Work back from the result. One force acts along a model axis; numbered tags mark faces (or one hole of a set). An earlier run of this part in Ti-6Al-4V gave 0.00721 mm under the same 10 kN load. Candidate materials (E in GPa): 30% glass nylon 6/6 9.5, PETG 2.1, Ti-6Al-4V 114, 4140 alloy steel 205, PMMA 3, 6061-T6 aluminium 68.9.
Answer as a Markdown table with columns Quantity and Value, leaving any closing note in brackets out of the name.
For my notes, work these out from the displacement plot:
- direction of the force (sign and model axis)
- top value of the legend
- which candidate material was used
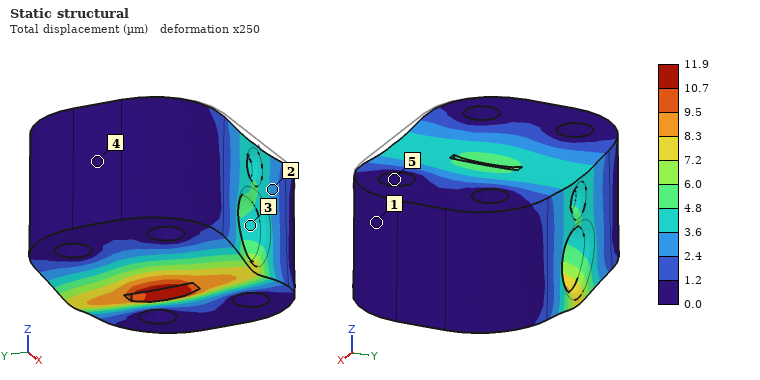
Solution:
| Quantity | Value |
|---|---|
| direction of the force | -Z |
| top value of the legend | 11.9 µm |
| which candidate material was used | 6061-T6 aluminium |
